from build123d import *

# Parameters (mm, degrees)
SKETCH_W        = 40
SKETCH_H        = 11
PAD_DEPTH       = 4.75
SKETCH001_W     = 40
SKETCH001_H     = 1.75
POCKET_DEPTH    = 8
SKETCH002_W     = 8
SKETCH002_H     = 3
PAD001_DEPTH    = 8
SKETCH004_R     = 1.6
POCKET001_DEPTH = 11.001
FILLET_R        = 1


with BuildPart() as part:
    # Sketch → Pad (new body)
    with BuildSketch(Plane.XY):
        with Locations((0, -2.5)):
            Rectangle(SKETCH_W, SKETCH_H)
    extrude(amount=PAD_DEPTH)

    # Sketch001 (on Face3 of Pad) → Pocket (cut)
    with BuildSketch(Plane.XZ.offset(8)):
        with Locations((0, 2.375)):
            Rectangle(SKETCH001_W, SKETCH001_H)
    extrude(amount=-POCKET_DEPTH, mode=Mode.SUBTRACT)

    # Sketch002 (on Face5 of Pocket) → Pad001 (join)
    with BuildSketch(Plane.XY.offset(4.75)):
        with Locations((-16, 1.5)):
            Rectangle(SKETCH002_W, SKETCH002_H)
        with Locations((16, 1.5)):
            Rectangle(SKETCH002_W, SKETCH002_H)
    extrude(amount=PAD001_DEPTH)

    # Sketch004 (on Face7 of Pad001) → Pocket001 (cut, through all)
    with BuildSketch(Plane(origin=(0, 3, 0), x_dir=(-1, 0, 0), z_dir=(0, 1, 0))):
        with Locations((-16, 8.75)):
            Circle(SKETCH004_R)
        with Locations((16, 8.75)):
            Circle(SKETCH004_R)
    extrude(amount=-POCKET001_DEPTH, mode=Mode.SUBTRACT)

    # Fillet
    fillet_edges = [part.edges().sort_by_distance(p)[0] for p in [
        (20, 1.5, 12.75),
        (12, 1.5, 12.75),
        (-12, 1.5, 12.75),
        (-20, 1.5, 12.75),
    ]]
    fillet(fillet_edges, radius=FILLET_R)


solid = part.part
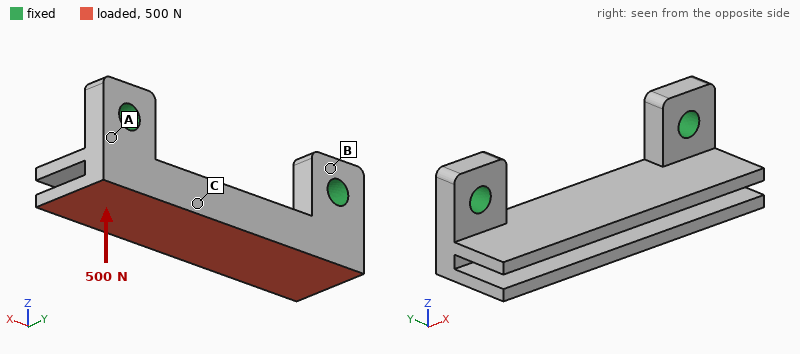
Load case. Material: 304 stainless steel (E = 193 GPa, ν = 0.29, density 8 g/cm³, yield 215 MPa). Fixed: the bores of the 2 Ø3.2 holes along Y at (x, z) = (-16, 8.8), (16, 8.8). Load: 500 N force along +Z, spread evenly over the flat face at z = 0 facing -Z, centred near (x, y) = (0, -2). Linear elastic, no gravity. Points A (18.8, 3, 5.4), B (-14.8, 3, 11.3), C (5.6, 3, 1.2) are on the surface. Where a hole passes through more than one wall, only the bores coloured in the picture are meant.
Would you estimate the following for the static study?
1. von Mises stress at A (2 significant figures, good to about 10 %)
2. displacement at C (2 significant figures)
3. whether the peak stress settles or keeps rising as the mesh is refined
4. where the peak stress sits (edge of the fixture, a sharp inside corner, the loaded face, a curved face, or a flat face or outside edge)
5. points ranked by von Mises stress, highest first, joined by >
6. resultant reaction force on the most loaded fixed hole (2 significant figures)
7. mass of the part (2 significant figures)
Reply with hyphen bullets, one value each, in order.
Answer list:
- 65 MPa
- 7.8 µm
- keeps rising
- edge of the fixture
- A > C > B
- 280 N
- 15 g
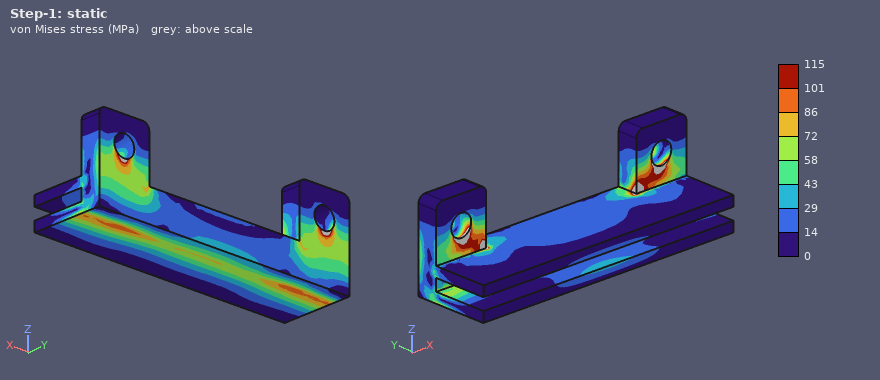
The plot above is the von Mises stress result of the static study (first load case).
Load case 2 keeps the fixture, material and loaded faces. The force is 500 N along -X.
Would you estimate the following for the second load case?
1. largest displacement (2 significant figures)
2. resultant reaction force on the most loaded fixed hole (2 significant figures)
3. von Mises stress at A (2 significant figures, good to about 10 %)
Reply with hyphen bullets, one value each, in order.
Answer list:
- 4.1 µm
- 260 N
- 20 MPa
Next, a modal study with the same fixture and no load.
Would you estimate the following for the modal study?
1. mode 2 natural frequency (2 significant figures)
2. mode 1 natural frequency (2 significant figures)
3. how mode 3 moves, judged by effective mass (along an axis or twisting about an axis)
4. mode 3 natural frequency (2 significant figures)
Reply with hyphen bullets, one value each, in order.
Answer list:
- 12 kHz
- 7400 Hz
- along Y
- 15 kHz
